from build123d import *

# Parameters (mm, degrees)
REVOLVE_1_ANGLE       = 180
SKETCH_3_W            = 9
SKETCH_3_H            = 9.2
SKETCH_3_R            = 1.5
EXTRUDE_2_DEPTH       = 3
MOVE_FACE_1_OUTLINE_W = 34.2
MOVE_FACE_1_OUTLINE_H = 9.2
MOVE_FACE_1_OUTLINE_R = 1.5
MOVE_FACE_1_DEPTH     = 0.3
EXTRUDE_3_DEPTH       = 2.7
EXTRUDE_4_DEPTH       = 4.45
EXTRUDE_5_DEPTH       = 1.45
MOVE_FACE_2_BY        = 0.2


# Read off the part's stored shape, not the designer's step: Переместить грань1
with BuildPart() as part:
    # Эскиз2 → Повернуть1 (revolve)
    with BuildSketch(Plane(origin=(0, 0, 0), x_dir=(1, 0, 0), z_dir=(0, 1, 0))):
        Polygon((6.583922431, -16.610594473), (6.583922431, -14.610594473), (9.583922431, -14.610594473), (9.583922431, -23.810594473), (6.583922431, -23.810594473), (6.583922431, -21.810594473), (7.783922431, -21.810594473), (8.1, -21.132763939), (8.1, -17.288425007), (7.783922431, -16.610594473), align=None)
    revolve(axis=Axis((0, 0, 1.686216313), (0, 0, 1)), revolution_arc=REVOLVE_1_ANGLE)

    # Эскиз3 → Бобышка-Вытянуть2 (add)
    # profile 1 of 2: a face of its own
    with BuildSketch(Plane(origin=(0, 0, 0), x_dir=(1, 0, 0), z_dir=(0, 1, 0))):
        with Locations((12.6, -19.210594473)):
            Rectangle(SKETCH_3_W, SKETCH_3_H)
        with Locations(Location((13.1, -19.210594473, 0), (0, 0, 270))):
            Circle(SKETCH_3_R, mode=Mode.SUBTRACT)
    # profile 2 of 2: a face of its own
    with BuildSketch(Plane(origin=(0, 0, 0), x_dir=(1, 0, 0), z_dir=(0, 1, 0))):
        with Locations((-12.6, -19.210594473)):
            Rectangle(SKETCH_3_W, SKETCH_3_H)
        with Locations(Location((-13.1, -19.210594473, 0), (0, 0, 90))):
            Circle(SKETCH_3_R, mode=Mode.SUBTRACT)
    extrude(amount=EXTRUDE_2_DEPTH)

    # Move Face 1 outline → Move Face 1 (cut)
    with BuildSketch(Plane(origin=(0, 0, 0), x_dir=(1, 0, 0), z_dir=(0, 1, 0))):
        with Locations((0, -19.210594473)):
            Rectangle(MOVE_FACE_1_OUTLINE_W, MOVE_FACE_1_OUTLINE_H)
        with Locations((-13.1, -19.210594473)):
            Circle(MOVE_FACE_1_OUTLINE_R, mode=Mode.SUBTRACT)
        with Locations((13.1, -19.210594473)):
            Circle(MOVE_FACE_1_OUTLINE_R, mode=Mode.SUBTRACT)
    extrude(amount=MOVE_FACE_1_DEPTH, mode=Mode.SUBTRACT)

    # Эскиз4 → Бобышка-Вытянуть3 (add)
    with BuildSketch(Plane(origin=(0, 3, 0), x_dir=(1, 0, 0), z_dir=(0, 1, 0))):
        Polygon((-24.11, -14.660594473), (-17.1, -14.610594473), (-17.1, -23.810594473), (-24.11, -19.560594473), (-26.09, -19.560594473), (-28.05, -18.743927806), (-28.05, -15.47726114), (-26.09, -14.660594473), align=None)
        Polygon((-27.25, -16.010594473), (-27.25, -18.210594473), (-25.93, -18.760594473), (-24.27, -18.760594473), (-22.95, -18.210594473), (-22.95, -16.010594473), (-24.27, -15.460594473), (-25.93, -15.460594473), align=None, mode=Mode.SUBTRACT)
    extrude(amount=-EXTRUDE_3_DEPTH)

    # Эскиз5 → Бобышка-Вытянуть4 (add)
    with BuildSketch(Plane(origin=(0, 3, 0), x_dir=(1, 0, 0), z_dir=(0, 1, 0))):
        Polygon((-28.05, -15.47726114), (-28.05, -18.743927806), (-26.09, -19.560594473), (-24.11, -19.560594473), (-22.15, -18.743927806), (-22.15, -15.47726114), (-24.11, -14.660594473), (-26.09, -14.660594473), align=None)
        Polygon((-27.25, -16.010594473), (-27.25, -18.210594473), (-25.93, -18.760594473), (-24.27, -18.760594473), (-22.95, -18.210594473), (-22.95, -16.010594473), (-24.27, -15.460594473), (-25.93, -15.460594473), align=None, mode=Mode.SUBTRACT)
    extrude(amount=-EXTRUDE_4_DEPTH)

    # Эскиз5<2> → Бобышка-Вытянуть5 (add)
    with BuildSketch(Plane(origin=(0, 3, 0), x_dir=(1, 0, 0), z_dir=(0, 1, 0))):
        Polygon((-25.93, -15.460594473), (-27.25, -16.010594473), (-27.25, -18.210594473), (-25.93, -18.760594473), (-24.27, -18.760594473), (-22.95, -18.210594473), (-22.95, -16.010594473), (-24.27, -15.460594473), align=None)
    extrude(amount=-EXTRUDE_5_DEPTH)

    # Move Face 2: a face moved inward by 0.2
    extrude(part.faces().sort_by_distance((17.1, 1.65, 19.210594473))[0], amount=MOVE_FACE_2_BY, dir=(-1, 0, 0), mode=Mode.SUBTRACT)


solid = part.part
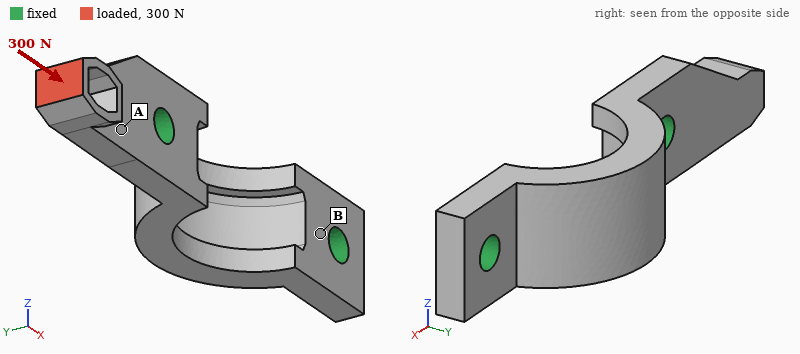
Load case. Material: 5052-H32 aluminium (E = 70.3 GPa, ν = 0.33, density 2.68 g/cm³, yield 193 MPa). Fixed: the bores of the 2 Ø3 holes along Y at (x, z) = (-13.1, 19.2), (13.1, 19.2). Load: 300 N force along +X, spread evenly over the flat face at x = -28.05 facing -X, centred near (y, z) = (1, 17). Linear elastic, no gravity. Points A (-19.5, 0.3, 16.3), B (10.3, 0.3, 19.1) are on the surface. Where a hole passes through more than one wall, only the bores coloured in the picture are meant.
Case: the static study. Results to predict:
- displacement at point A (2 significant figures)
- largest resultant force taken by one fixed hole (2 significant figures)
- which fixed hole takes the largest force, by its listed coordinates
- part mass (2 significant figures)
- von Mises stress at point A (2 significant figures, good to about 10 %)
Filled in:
7.3 µm
300 N
(-13.1, 19.2)
2.8 g
52 MPa
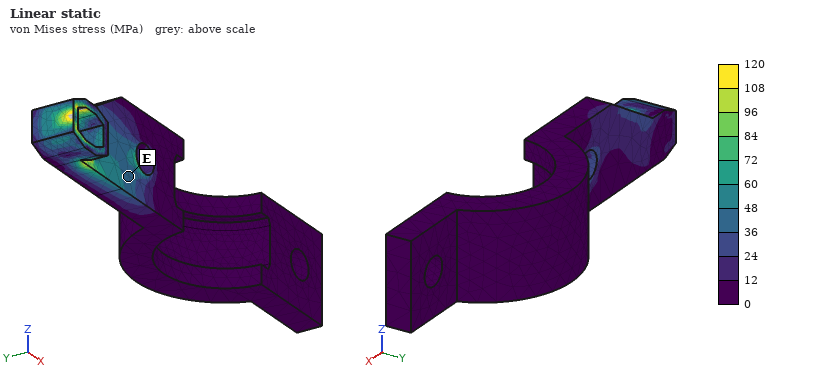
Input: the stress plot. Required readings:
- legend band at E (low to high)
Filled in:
36 to 48 MPa
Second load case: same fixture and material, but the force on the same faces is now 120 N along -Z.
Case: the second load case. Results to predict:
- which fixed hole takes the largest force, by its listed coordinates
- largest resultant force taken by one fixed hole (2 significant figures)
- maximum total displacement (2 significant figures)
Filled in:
(-13.1, 19.2)
130 N
43 µm
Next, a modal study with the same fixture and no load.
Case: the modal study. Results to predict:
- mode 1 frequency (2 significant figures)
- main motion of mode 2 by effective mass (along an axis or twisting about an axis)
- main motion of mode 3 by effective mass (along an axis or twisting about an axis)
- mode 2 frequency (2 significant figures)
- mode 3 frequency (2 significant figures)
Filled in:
13 kHz
along Z
along Z
18 kHz
26 kHz
